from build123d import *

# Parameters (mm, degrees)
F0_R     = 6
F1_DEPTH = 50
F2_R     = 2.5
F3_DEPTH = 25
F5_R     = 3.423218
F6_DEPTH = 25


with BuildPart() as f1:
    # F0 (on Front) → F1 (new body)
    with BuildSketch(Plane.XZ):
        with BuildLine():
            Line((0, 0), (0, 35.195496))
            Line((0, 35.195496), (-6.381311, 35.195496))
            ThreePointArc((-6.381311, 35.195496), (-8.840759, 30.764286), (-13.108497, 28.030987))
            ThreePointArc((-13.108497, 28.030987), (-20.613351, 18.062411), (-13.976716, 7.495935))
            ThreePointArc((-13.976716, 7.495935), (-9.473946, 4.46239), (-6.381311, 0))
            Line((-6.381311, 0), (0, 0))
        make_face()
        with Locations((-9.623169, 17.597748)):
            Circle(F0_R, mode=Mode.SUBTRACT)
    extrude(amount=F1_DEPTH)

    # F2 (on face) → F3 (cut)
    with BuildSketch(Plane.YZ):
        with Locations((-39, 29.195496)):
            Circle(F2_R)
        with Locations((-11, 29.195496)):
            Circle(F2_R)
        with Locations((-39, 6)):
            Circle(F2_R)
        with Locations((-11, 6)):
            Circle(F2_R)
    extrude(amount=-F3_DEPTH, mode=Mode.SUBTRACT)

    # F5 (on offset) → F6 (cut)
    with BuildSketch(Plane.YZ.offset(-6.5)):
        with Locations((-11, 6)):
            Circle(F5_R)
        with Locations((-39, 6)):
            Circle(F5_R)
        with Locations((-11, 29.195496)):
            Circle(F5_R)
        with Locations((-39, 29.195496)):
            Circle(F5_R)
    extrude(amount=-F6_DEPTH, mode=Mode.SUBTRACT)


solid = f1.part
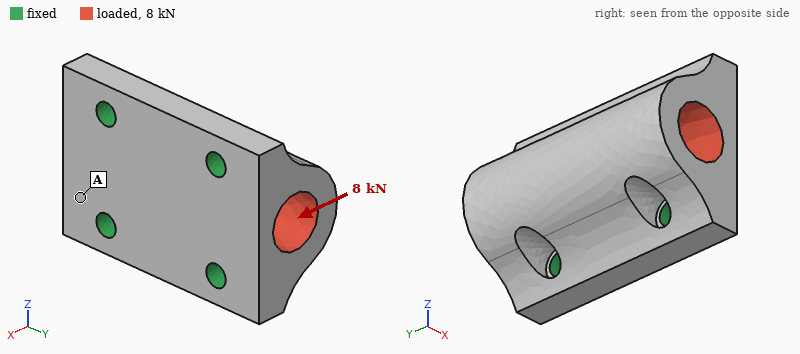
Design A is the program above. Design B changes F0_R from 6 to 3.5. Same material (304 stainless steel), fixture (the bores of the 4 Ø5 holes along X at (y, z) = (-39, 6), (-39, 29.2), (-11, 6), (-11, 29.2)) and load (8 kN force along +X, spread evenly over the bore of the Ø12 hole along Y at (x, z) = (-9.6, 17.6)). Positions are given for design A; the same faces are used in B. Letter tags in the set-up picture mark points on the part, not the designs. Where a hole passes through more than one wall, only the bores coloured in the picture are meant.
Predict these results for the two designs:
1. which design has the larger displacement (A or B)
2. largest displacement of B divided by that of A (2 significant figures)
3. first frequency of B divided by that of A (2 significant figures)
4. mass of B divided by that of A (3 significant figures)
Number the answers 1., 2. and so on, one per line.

1. A
2. 0.84
3. 0.98
4. 1.20
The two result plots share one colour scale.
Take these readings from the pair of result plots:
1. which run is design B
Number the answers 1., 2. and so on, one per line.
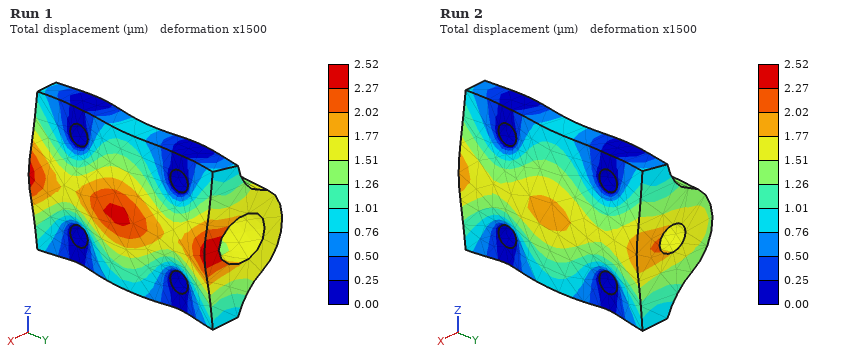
1. Run 2
